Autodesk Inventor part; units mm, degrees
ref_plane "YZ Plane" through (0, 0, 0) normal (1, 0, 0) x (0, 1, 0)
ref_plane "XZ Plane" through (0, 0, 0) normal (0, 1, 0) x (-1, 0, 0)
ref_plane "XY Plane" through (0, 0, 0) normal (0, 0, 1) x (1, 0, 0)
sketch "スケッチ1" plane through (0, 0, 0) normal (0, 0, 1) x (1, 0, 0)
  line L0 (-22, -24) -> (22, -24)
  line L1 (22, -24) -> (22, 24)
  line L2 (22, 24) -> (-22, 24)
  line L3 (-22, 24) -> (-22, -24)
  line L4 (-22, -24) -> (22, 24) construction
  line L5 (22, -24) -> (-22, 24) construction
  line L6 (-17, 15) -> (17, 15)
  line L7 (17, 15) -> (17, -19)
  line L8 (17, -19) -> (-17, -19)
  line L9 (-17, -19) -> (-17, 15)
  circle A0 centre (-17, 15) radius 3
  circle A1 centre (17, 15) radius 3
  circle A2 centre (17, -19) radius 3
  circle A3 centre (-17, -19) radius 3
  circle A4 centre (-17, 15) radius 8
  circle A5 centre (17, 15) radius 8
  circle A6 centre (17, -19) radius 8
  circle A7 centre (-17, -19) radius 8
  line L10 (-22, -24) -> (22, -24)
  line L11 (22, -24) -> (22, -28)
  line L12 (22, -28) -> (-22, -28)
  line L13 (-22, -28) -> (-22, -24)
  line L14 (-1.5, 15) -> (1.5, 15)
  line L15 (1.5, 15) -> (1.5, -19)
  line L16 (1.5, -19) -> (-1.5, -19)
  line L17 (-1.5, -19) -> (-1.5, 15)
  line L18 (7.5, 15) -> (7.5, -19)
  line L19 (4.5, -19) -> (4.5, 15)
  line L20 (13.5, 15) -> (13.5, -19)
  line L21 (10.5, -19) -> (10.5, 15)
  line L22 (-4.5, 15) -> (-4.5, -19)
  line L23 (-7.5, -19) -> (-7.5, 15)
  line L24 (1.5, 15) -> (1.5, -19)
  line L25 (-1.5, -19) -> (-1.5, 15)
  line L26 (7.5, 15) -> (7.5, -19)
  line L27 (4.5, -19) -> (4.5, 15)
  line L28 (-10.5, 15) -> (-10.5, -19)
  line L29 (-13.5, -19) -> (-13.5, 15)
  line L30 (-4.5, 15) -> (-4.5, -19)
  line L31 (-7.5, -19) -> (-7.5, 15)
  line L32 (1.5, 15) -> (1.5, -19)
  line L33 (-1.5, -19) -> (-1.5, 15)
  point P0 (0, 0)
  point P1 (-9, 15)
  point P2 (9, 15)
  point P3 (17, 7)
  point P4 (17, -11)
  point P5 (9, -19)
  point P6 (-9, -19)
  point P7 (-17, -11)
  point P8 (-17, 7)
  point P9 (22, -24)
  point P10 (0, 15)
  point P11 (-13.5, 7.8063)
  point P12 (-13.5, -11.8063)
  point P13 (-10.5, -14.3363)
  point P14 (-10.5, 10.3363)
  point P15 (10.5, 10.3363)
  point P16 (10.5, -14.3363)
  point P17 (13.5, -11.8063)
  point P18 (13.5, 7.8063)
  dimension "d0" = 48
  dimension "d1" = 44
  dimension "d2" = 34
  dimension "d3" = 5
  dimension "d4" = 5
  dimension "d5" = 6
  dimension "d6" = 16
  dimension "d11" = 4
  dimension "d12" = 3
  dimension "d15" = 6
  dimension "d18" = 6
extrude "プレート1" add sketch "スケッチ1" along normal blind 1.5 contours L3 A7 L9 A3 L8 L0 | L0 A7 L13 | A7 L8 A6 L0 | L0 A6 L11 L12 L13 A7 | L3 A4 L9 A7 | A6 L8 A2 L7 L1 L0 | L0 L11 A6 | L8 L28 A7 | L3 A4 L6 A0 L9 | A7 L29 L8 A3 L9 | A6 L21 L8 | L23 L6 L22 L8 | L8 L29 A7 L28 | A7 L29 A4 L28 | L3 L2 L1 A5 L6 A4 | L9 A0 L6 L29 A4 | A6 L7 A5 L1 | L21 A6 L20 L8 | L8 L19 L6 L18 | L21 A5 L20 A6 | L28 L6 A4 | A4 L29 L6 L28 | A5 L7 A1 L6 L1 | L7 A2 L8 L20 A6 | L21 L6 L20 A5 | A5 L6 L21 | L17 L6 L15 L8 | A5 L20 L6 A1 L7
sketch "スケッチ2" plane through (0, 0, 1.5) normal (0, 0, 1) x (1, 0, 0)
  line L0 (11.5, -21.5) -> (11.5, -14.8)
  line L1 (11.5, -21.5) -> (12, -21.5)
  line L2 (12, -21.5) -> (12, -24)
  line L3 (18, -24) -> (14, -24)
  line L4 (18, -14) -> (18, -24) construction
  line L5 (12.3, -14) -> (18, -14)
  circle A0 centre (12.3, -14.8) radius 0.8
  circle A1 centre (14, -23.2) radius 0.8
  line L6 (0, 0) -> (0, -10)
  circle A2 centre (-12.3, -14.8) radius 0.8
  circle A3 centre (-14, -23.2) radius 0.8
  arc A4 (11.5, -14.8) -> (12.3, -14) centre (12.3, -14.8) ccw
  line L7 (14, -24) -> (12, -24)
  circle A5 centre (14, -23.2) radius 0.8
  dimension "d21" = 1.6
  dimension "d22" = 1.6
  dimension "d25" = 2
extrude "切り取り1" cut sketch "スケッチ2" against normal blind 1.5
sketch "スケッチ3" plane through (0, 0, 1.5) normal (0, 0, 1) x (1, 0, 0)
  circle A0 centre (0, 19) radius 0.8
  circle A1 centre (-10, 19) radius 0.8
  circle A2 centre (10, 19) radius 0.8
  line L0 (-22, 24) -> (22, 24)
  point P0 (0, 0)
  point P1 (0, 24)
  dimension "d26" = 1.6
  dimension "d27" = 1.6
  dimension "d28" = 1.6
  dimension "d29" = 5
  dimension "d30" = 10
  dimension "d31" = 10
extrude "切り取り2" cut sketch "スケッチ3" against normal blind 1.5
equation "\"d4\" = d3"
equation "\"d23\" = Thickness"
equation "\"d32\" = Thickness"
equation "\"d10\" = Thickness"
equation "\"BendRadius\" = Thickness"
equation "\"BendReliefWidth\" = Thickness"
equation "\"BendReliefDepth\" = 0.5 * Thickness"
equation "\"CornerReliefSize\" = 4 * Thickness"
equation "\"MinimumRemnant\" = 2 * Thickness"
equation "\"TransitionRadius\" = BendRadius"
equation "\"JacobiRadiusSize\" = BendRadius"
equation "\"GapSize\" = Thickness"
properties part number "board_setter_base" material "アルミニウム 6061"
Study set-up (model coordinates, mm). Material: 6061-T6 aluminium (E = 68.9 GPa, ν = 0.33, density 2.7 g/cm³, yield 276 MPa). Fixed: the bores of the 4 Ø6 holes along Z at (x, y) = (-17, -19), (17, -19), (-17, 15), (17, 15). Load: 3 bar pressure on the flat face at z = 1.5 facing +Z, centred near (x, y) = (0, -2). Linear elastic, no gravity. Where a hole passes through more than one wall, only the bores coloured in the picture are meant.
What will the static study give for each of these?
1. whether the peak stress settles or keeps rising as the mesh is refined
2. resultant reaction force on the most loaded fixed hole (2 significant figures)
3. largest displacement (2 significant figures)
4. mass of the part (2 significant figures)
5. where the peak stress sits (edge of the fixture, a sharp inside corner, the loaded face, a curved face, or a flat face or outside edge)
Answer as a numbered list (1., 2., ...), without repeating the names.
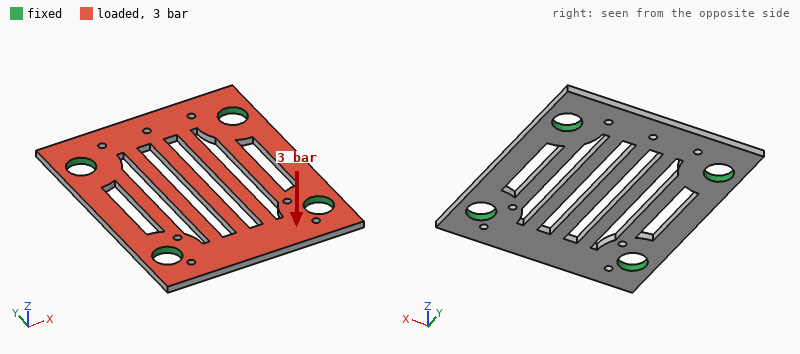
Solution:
1. keeps rising
2. 120 N
3. 0.18 mm
4. 6.7 g
5. edge of the fixture
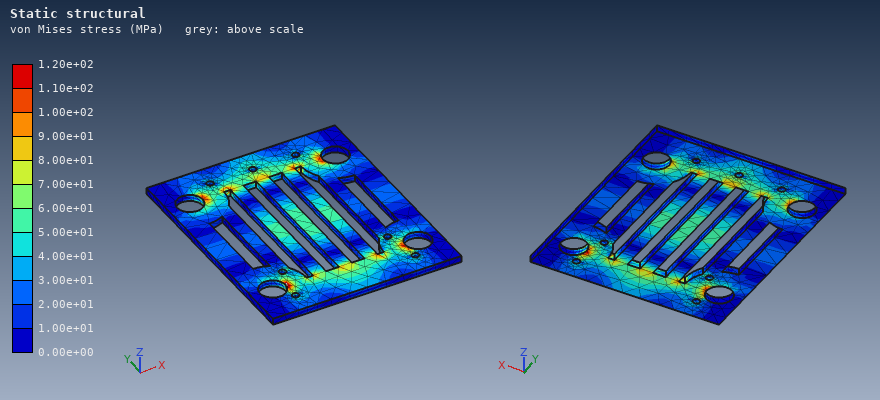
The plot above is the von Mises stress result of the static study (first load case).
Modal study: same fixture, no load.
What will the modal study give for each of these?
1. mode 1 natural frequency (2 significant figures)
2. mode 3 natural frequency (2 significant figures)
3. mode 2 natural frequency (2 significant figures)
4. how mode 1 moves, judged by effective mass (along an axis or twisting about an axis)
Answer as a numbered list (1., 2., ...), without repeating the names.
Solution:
1. 3900 Hz
2. 5400 Hz
3. 5100 Hz
4. along Z
